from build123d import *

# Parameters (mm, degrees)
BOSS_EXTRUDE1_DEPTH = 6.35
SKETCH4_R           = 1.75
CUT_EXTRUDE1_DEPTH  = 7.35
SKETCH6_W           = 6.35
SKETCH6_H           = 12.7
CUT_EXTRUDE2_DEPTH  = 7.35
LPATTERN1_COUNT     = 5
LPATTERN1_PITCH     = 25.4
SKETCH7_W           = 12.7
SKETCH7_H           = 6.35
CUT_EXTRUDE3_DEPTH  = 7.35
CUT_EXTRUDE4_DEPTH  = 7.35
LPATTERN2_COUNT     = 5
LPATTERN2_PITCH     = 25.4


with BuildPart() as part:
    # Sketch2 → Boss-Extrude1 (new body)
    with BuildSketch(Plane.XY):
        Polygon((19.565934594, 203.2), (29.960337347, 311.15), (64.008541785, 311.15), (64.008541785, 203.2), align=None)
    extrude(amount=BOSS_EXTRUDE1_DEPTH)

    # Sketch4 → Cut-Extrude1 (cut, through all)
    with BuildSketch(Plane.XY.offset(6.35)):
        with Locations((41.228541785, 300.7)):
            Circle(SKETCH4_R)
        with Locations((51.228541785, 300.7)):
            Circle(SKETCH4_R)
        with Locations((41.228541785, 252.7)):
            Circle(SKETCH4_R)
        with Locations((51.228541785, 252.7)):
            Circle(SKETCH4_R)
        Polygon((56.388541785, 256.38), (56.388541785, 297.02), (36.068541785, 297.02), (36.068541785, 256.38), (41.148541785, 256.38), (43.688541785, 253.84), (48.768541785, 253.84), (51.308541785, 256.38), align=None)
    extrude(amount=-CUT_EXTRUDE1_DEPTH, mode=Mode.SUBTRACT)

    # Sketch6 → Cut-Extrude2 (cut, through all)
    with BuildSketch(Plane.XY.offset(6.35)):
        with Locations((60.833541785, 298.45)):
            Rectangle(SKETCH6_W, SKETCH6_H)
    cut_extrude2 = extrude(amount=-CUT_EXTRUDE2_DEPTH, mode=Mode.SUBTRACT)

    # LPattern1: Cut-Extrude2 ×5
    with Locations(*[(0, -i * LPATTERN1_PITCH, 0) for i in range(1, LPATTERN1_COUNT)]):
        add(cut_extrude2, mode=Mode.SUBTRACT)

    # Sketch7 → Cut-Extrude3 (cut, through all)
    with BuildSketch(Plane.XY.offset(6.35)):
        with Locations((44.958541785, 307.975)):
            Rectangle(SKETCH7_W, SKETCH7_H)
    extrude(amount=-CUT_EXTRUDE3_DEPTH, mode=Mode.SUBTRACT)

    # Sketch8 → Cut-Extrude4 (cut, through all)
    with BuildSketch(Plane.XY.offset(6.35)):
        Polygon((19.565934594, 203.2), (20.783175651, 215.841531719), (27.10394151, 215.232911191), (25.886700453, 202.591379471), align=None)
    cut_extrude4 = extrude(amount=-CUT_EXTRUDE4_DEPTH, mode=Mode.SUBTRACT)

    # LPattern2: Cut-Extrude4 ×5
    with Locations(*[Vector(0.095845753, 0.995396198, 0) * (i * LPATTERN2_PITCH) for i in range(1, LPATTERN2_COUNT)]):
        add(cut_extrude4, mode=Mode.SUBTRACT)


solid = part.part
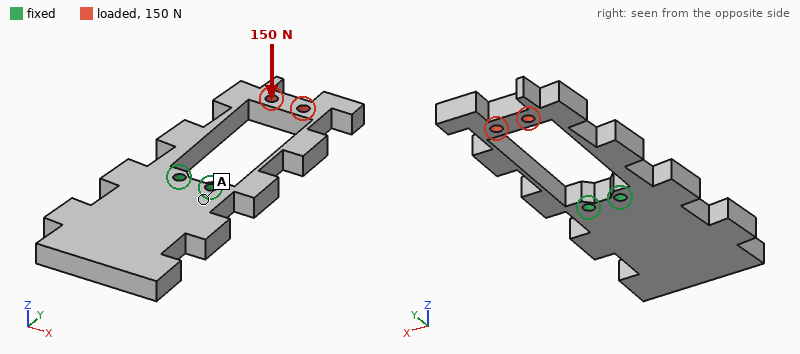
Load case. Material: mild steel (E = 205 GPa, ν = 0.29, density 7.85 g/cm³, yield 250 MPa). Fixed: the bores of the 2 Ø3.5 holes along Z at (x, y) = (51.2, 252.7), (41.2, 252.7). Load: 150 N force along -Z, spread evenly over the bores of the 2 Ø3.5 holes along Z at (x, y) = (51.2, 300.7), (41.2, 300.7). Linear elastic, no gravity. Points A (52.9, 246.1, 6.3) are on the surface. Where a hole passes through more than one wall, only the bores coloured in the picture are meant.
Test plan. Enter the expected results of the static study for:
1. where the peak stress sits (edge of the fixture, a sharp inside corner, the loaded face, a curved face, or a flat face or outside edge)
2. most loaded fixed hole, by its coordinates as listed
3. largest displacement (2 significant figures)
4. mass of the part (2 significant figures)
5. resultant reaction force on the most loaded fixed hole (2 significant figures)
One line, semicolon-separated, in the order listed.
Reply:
a flat face or outside edge; (51.2, 252.7); 0.31 mm; 130 g; 85 N
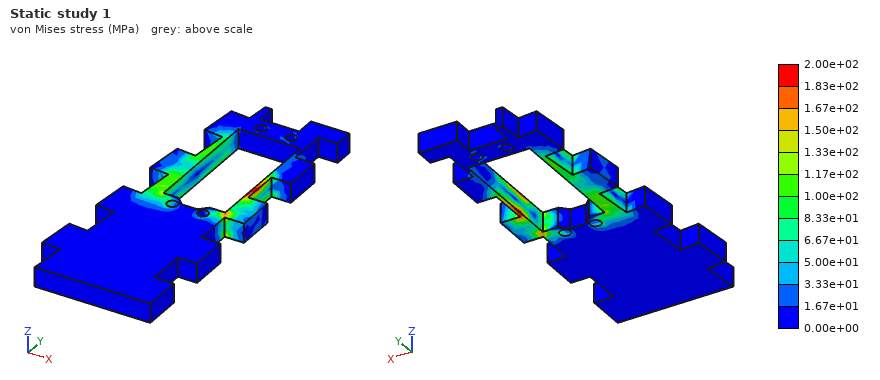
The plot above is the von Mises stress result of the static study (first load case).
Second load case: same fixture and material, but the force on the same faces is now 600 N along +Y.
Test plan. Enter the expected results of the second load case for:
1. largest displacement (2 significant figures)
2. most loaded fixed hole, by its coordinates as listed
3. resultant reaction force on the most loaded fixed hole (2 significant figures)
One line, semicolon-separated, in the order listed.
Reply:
22 µm; (41.2, 252.7); 340 N
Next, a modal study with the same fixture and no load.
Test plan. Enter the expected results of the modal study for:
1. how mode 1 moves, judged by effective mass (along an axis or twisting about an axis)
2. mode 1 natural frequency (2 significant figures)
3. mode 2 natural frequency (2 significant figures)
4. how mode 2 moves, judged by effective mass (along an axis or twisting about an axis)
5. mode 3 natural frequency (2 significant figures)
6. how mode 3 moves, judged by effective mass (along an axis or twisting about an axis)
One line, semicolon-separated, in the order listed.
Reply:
along Z; 900 Hz; 1100 Hz; along X; 1800 Hz; along Z
